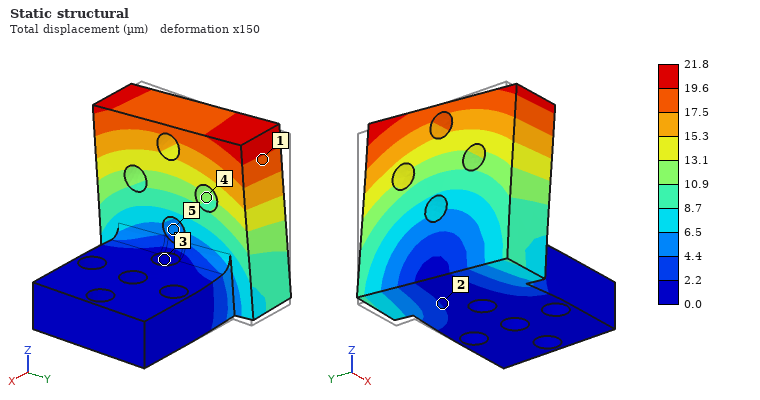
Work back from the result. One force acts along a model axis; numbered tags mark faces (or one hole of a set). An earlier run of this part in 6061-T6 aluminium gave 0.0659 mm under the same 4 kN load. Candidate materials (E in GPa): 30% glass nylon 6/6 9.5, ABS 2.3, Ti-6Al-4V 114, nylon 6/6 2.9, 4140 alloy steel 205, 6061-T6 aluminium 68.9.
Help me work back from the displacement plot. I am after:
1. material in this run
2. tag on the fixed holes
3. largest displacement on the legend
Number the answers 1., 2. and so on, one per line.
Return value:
1. 4140 alloy steel
2. 3
3. 21.8 µm
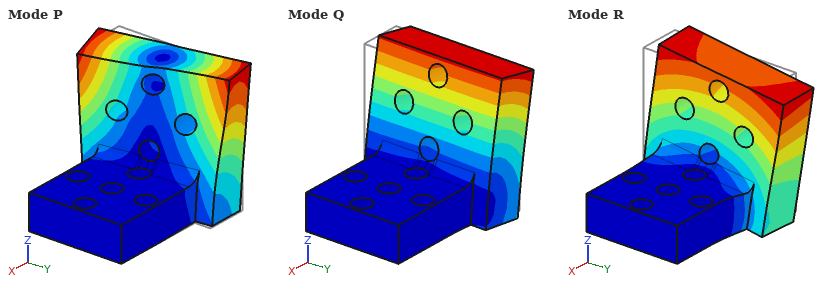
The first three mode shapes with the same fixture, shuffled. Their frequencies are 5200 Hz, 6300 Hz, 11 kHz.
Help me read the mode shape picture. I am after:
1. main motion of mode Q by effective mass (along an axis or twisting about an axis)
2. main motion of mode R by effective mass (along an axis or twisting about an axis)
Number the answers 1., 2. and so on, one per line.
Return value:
1. along X
2. along Y
